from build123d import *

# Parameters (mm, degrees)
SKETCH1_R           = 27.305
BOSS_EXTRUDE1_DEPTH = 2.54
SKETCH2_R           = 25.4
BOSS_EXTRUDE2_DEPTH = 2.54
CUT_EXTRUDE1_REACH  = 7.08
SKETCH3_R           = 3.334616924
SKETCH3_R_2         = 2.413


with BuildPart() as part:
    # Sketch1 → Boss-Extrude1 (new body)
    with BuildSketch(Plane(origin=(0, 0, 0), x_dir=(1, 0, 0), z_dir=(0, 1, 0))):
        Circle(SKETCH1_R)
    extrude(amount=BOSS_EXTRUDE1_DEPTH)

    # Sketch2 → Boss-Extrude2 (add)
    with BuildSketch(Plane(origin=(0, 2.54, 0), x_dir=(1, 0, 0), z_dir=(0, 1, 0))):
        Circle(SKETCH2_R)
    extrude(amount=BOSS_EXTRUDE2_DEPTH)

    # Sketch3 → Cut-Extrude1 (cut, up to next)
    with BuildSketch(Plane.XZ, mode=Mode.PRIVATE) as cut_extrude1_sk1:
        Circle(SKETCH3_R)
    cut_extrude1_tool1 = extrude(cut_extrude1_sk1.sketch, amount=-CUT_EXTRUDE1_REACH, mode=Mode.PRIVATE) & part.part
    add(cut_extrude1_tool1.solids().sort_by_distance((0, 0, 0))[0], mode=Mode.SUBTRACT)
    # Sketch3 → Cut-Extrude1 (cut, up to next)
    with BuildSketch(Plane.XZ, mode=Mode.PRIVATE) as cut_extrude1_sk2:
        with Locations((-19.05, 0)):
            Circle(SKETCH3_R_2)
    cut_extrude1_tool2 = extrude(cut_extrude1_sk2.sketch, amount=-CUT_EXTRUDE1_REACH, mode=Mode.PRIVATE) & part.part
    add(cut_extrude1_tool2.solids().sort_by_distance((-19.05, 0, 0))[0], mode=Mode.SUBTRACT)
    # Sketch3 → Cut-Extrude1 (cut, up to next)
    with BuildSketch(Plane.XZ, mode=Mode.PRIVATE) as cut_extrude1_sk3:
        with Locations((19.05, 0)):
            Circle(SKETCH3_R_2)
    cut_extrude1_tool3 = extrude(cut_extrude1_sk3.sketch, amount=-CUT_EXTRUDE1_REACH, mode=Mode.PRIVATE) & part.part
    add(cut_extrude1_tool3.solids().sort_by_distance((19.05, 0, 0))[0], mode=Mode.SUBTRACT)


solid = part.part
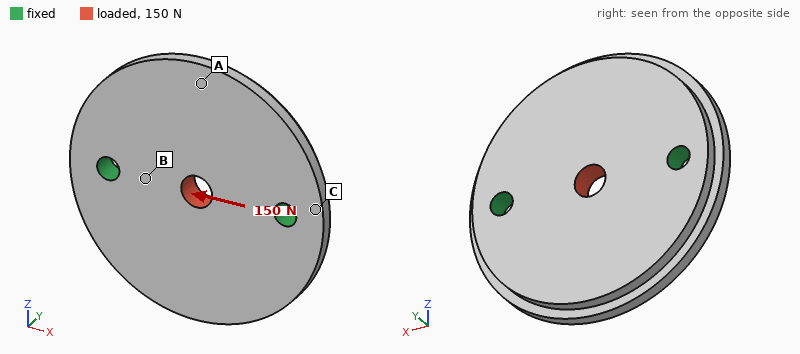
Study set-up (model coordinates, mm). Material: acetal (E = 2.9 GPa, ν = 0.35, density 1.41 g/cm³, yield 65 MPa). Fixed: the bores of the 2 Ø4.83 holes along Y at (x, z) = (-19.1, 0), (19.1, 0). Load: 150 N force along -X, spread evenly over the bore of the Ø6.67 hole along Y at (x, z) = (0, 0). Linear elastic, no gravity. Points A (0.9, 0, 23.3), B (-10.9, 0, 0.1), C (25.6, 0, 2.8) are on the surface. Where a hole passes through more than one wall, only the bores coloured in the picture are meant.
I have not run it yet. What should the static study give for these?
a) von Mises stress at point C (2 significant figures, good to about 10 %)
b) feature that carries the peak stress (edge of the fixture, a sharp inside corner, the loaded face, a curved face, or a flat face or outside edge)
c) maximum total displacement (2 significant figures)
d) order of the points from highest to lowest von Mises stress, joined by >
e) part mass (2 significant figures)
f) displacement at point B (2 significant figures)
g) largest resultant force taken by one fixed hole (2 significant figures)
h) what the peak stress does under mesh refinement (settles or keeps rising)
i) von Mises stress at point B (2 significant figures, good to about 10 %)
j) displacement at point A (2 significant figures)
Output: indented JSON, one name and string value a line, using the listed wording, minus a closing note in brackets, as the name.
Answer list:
{
  "von Mises stress at point C": "0.35 MPa",
  "feature that carries the peak stress": "edge of the fixture",
  "maximum total displacement": "6.7 µm",
  "order of the points from highest to lowest von Mises stress, joined by >": "B > C > A",
  "part mass": "15 g",
  "displacement at point B": "2.8 µm",
  "largest resultant force taken by one fixed hole": "75 N",
  "what the peak stress does under mesh refinement": "keeps rising",
  "von Mises stress at point B": "1.3 MPa",
  "displacement at point A": "2.5 µm"
}
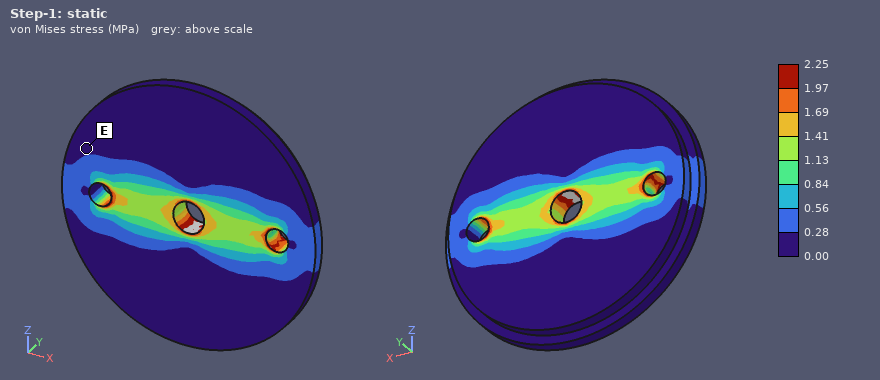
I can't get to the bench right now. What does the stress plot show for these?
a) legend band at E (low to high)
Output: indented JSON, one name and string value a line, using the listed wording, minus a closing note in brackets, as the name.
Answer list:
{
  "legend band at E": "0.00 to 0.28 MPa"
}
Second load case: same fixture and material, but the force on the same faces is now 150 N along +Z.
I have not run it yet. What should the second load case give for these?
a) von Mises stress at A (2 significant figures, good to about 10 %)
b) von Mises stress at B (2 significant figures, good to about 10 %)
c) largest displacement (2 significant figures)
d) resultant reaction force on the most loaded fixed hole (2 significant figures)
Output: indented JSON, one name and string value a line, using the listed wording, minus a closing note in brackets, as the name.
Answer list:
{
  "von Mises stress at A": "0.43 MPa",
  "von Mises stress at B": "0.59 MPa",
  "largest displacement": "9.8 µm",
  "resultant reaction force on the most loaded fixed hole": "75 N"
}
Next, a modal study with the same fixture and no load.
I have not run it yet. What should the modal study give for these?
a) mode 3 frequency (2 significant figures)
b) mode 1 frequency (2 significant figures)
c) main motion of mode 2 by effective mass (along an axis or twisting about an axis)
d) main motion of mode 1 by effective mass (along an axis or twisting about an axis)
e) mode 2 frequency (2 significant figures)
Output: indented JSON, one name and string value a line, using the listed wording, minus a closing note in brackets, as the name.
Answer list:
{
  "mode 3 frequency": "4200 Hz",
  "mode 1 frequency": "1600 Hz",
  "main motion of mode 2 by effective mass": "along Y",
  "main motion of mode 1 by effective mass": "twisting about X",
  "mode 2 frequency": "2000 Hz"
}
